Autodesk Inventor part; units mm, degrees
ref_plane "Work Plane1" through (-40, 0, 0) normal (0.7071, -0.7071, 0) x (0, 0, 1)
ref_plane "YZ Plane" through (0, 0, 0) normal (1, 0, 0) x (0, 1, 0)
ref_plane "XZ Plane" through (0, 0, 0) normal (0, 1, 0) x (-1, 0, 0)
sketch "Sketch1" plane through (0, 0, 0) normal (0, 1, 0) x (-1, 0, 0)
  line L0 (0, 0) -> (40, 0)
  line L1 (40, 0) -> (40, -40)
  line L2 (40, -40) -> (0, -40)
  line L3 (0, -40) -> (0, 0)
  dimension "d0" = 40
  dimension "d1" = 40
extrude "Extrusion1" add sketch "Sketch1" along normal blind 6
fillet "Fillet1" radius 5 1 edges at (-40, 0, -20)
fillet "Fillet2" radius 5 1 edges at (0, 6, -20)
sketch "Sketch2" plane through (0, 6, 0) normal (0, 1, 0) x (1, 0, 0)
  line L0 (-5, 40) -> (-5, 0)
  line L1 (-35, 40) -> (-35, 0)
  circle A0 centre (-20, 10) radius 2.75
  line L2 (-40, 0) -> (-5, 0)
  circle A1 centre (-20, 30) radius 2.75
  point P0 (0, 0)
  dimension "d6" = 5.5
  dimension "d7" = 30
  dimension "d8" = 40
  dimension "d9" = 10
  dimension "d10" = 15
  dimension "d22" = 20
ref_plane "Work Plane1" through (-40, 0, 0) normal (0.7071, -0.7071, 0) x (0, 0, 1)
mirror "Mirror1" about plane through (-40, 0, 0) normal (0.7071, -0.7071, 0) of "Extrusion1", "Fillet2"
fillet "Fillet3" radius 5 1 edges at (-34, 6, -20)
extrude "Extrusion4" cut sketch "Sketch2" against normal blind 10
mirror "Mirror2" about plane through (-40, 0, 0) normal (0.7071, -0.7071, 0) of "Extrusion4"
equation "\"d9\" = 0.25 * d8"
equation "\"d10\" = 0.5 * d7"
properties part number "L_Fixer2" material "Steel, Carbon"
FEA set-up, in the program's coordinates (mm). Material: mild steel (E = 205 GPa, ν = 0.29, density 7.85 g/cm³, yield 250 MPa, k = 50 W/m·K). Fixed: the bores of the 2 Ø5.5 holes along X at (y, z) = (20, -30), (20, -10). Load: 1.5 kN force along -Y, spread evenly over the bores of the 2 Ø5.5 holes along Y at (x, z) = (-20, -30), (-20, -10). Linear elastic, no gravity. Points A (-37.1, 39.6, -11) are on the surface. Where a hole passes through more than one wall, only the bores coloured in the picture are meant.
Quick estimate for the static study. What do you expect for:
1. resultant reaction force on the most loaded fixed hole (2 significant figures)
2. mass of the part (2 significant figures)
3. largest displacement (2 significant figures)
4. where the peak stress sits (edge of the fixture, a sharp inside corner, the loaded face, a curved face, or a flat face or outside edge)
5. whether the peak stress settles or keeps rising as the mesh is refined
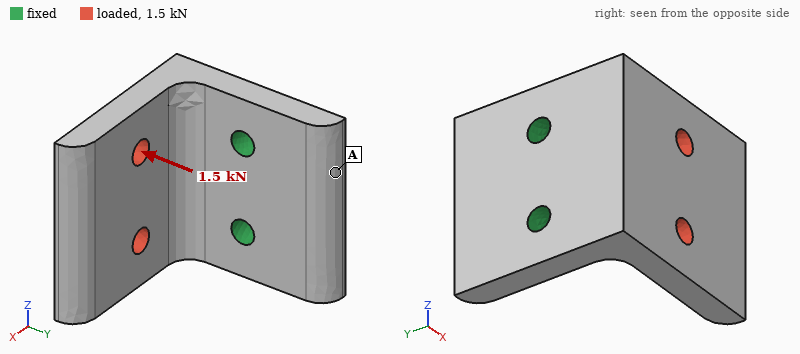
770 N
130 g
0.11 mm
edge of the fixture
keeps rising
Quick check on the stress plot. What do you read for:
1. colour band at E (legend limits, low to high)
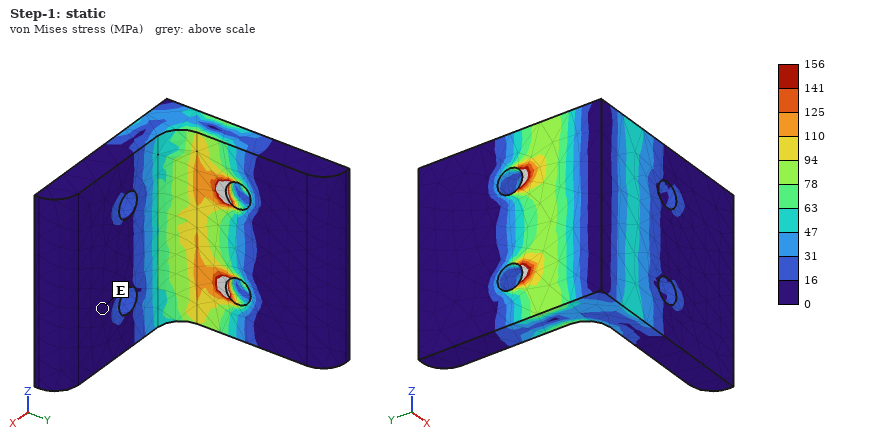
0 to 16 MPa
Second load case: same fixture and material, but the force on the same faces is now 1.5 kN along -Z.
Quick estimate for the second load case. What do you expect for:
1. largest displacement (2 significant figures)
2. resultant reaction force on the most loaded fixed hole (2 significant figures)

29 µm
1.6 kN
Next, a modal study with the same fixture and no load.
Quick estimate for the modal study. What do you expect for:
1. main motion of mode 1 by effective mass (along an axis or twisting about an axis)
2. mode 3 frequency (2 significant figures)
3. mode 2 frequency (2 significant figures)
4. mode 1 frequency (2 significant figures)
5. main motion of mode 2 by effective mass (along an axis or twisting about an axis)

along Y
8000 Hz
4800 Hz
2500 Hz
along Z
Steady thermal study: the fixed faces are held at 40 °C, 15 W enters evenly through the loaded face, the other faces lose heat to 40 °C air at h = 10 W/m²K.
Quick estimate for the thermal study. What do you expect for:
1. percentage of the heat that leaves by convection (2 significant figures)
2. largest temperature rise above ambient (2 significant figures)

7.9 %
38 K
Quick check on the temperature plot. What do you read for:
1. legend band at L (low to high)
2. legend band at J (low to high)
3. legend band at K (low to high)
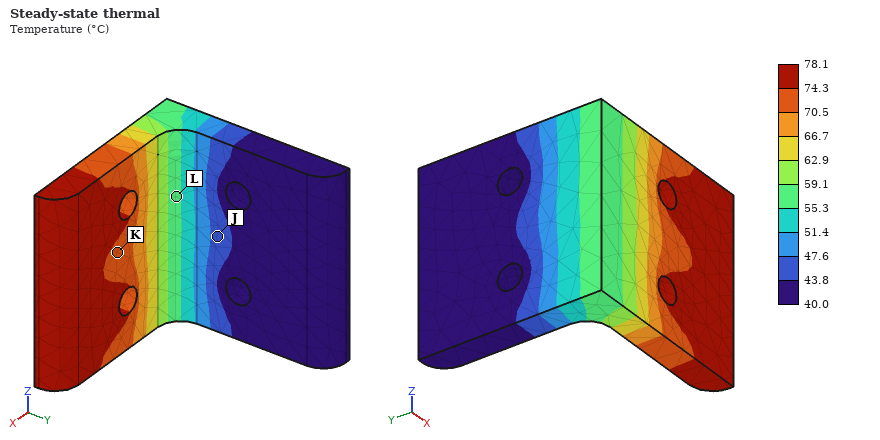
55.3 to 59.1 °C
43.8 to 47.6 °C
70.5 to 74.3 °C
